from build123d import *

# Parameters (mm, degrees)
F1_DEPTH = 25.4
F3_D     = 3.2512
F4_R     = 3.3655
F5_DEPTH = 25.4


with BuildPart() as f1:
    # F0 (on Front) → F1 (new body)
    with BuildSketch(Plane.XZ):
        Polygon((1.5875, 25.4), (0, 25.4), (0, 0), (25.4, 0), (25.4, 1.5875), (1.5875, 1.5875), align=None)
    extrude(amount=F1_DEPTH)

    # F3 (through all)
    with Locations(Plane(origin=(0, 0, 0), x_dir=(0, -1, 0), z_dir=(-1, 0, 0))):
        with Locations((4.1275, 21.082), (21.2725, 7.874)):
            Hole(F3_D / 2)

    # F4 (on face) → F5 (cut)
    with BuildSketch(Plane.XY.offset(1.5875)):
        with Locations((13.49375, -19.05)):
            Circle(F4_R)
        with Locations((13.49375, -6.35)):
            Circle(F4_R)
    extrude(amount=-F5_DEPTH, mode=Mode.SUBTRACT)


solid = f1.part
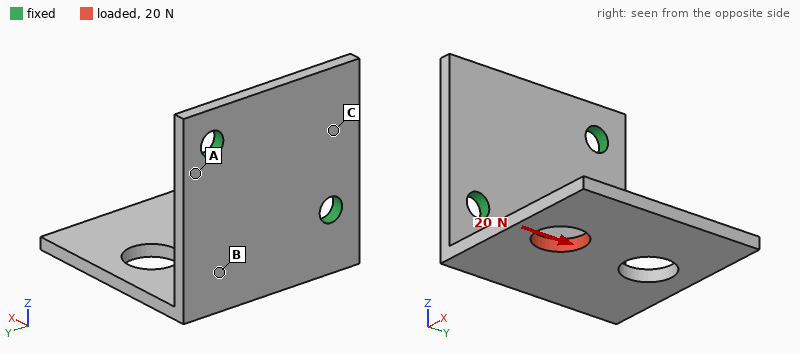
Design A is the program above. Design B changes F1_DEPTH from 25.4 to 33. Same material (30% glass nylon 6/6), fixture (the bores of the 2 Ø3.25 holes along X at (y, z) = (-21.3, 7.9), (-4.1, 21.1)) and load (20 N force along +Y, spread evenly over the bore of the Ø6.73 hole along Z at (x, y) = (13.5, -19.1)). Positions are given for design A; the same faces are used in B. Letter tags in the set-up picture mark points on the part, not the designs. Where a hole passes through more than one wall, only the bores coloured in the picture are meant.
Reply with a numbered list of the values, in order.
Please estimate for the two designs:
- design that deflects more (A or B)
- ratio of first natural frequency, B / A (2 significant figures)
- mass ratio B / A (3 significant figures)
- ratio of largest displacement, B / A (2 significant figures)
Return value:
1. A
2. 1.0
3. 1.32
4. 0.71
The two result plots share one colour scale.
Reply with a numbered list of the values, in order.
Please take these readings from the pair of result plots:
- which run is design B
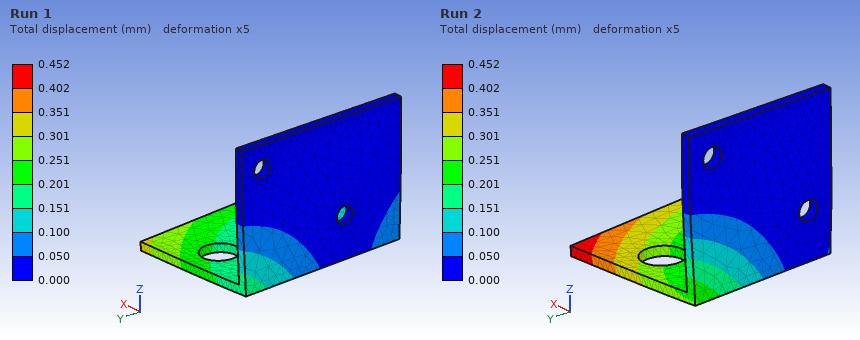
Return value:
1. Run 1
